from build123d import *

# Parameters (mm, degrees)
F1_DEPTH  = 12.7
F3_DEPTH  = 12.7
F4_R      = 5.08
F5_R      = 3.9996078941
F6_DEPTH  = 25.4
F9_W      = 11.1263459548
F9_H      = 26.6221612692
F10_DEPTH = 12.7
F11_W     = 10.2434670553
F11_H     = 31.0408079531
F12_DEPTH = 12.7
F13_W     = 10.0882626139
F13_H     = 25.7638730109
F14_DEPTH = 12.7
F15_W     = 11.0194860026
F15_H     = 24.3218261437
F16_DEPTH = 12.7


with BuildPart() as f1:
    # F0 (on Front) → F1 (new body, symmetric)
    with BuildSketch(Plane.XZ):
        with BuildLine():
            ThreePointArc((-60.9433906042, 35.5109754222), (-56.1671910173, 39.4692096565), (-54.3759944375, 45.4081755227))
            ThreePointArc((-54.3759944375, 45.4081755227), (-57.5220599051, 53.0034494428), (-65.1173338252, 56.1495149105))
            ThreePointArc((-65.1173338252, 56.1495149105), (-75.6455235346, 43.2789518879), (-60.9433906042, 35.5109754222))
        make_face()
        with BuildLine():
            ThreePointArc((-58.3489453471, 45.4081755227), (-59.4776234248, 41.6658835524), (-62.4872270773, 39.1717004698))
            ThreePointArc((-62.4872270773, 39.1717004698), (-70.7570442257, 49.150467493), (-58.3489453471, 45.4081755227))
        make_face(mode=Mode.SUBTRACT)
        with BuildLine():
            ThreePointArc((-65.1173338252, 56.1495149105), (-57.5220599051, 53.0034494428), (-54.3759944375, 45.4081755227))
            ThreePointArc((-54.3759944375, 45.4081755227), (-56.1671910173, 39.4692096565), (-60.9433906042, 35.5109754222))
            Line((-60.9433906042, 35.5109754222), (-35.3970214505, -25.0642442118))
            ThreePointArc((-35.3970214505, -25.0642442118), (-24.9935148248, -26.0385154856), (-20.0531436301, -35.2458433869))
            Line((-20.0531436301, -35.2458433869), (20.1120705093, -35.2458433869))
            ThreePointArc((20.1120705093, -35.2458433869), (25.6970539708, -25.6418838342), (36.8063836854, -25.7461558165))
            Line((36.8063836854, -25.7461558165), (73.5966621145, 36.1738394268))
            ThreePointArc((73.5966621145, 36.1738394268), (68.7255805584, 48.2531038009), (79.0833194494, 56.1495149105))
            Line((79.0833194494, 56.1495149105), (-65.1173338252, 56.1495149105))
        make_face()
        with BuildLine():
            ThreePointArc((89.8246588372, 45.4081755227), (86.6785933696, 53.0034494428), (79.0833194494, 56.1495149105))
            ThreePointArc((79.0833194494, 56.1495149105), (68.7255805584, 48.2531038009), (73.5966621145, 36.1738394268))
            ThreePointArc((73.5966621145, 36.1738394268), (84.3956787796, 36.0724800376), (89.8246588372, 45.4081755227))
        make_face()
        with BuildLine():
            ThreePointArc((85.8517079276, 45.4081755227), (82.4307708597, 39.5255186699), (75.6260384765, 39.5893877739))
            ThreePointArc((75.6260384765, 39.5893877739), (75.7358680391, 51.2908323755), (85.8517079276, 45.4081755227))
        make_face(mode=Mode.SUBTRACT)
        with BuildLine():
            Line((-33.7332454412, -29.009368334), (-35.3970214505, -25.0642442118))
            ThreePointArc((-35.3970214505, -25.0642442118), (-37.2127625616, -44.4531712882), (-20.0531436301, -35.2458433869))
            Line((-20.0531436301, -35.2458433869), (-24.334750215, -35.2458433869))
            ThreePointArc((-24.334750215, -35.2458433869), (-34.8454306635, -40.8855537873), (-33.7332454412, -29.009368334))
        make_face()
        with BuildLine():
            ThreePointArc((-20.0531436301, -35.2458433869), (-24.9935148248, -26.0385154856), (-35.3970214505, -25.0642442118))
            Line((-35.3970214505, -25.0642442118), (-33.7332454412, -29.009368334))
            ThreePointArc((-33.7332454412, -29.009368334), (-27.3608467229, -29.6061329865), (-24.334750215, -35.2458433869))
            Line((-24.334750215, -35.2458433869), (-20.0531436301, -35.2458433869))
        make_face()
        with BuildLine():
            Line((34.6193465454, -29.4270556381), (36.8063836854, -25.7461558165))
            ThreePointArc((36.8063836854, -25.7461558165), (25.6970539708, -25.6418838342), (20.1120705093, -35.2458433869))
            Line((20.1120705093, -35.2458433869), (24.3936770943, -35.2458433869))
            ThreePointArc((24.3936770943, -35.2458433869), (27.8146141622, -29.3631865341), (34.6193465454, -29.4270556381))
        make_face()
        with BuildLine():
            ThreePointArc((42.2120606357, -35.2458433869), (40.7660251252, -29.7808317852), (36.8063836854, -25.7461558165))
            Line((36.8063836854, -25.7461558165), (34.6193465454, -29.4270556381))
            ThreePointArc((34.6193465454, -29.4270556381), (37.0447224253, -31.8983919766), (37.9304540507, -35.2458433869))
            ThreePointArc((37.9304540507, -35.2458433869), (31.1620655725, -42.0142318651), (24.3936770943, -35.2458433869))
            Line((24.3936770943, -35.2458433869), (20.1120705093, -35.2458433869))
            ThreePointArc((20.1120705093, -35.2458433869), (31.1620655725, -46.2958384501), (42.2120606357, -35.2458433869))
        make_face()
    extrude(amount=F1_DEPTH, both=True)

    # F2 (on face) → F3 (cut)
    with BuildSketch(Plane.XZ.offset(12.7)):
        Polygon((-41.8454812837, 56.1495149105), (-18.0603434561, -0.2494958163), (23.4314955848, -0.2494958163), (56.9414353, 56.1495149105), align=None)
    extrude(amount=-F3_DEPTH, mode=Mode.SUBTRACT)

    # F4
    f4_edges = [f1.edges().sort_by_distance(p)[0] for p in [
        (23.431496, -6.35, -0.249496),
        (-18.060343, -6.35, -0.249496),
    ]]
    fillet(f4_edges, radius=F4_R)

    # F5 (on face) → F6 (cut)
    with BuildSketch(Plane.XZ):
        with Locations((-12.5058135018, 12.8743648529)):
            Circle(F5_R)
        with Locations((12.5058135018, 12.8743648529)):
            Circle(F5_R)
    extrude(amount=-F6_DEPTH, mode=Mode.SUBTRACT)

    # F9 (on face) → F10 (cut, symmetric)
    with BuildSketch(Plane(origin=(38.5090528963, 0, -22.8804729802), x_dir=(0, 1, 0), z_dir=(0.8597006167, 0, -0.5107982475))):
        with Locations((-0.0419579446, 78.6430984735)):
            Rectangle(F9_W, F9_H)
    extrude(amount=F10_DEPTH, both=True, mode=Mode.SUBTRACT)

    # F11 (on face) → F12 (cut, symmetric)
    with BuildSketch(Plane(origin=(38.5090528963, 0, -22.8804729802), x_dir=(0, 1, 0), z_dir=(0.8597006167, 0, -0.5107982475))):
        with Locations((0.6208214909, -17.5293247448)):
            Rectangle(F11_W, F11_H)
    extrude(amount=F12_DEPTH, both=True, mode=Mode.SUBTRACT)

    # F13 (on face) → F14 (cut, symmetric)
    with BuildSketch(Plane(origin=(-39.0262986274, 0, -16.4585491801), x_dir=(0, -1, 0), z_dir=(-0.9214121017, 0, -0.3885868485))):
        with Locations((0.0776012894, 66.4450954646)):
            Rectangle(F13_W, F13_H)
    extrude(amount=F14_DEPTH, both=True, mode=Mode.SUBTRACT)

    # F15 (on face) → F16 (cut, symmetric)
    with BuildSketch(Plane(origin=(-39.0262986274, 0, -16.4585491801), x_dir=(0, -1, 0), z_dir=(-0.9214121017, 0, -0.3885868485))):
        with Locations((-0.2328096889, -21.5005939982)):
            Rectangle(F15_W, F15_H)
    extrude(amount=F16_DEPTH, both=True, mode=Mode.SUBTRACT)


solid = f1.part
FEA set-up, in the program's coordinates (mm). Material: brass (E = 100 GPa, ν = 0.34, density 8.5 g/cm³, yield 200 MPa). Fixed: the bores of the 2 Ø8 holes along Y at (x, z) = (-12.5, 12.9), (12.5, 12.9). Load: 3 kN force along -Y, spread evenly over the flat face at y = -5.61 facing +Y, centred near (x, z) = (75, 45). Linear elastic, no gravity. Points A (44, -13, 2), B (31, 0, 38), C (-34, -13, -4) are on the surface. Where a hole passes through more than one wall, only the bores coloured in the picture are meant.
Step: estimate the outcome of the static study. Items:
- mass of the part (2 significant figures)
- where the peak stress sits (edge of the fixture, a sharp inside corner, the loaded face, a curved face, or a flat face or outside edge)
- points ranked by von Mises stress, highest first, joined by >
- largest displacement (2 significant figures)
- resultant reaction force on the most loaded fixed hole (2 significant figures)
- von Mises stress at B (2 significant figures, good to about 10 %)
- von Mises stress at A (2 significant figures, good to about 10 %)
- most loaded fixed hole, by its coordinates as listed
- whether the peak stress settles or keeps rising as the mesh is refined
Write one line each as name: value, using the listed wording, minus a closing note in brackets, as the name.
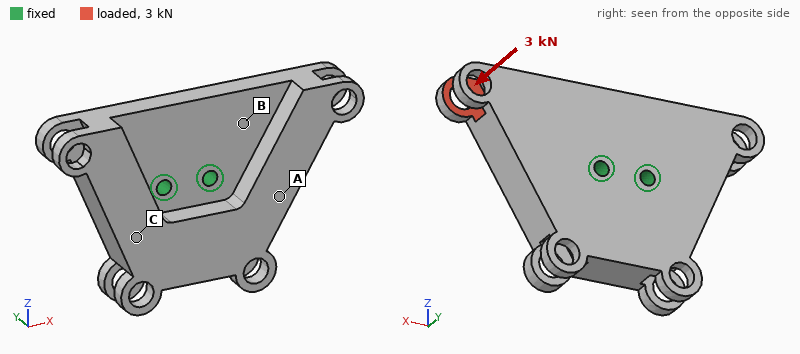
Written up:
mass of the part: 1.7 kg
where the peak stress sits: edge of the fixture
points ranked by von Mises stress, highest first, joined by >: A > B > C
largest displacement: 0.34 mm
resultant reaction force on the most loaded fixed hole: 6.8 kN
von Mises stress at B: 27 MPa
von Mises stress at A: 41 MPa
most loaded fixed hole, by its coordinates as listed: (12.5, 12.9)
whether the peak stress settles or keeps rising as the mesh is refined: keeps rising
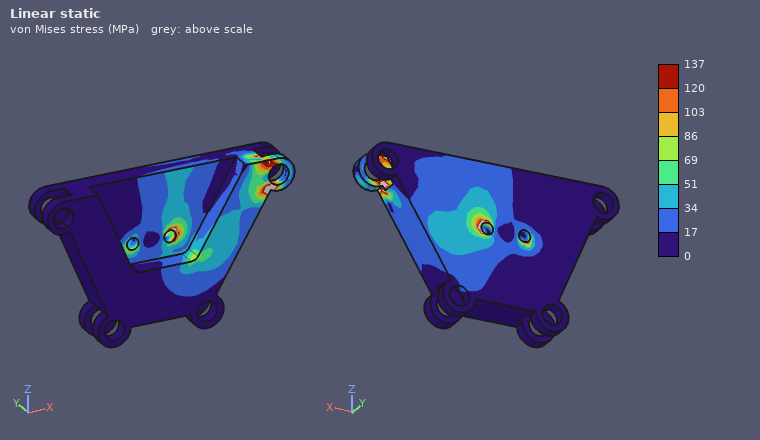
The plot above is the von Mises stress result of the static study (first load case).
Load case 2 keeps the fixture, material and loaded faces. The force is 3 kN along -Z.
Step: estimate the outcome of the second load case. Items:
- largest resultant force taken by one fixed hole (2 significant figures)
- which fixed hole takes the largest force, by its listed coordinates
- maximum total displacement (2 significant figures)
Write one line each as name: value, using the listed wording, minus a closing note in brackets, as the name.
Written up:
largest resultant force taken by one fixed hole: 8.7 kN
which fixed hole takes the largest force, by its listed coordinates: (12.5, 12.9)
maximum total displacement: 0.11 mm
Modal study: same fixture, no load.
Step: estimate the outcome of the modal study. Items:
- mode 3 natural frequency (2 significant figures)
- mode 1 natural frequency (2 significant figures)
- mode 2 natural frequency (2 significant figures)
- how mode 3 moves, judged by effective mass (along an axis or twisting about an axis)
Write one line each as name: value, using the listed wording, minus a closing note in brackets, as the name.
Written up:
mode 3 natural frequency: 2500 Hz
mode 1 natural frequency: 1600 Hz
mode 2 natural frequency: 1900 Hz
how mode 3 moves, judged by effective mass: twisting about Y
